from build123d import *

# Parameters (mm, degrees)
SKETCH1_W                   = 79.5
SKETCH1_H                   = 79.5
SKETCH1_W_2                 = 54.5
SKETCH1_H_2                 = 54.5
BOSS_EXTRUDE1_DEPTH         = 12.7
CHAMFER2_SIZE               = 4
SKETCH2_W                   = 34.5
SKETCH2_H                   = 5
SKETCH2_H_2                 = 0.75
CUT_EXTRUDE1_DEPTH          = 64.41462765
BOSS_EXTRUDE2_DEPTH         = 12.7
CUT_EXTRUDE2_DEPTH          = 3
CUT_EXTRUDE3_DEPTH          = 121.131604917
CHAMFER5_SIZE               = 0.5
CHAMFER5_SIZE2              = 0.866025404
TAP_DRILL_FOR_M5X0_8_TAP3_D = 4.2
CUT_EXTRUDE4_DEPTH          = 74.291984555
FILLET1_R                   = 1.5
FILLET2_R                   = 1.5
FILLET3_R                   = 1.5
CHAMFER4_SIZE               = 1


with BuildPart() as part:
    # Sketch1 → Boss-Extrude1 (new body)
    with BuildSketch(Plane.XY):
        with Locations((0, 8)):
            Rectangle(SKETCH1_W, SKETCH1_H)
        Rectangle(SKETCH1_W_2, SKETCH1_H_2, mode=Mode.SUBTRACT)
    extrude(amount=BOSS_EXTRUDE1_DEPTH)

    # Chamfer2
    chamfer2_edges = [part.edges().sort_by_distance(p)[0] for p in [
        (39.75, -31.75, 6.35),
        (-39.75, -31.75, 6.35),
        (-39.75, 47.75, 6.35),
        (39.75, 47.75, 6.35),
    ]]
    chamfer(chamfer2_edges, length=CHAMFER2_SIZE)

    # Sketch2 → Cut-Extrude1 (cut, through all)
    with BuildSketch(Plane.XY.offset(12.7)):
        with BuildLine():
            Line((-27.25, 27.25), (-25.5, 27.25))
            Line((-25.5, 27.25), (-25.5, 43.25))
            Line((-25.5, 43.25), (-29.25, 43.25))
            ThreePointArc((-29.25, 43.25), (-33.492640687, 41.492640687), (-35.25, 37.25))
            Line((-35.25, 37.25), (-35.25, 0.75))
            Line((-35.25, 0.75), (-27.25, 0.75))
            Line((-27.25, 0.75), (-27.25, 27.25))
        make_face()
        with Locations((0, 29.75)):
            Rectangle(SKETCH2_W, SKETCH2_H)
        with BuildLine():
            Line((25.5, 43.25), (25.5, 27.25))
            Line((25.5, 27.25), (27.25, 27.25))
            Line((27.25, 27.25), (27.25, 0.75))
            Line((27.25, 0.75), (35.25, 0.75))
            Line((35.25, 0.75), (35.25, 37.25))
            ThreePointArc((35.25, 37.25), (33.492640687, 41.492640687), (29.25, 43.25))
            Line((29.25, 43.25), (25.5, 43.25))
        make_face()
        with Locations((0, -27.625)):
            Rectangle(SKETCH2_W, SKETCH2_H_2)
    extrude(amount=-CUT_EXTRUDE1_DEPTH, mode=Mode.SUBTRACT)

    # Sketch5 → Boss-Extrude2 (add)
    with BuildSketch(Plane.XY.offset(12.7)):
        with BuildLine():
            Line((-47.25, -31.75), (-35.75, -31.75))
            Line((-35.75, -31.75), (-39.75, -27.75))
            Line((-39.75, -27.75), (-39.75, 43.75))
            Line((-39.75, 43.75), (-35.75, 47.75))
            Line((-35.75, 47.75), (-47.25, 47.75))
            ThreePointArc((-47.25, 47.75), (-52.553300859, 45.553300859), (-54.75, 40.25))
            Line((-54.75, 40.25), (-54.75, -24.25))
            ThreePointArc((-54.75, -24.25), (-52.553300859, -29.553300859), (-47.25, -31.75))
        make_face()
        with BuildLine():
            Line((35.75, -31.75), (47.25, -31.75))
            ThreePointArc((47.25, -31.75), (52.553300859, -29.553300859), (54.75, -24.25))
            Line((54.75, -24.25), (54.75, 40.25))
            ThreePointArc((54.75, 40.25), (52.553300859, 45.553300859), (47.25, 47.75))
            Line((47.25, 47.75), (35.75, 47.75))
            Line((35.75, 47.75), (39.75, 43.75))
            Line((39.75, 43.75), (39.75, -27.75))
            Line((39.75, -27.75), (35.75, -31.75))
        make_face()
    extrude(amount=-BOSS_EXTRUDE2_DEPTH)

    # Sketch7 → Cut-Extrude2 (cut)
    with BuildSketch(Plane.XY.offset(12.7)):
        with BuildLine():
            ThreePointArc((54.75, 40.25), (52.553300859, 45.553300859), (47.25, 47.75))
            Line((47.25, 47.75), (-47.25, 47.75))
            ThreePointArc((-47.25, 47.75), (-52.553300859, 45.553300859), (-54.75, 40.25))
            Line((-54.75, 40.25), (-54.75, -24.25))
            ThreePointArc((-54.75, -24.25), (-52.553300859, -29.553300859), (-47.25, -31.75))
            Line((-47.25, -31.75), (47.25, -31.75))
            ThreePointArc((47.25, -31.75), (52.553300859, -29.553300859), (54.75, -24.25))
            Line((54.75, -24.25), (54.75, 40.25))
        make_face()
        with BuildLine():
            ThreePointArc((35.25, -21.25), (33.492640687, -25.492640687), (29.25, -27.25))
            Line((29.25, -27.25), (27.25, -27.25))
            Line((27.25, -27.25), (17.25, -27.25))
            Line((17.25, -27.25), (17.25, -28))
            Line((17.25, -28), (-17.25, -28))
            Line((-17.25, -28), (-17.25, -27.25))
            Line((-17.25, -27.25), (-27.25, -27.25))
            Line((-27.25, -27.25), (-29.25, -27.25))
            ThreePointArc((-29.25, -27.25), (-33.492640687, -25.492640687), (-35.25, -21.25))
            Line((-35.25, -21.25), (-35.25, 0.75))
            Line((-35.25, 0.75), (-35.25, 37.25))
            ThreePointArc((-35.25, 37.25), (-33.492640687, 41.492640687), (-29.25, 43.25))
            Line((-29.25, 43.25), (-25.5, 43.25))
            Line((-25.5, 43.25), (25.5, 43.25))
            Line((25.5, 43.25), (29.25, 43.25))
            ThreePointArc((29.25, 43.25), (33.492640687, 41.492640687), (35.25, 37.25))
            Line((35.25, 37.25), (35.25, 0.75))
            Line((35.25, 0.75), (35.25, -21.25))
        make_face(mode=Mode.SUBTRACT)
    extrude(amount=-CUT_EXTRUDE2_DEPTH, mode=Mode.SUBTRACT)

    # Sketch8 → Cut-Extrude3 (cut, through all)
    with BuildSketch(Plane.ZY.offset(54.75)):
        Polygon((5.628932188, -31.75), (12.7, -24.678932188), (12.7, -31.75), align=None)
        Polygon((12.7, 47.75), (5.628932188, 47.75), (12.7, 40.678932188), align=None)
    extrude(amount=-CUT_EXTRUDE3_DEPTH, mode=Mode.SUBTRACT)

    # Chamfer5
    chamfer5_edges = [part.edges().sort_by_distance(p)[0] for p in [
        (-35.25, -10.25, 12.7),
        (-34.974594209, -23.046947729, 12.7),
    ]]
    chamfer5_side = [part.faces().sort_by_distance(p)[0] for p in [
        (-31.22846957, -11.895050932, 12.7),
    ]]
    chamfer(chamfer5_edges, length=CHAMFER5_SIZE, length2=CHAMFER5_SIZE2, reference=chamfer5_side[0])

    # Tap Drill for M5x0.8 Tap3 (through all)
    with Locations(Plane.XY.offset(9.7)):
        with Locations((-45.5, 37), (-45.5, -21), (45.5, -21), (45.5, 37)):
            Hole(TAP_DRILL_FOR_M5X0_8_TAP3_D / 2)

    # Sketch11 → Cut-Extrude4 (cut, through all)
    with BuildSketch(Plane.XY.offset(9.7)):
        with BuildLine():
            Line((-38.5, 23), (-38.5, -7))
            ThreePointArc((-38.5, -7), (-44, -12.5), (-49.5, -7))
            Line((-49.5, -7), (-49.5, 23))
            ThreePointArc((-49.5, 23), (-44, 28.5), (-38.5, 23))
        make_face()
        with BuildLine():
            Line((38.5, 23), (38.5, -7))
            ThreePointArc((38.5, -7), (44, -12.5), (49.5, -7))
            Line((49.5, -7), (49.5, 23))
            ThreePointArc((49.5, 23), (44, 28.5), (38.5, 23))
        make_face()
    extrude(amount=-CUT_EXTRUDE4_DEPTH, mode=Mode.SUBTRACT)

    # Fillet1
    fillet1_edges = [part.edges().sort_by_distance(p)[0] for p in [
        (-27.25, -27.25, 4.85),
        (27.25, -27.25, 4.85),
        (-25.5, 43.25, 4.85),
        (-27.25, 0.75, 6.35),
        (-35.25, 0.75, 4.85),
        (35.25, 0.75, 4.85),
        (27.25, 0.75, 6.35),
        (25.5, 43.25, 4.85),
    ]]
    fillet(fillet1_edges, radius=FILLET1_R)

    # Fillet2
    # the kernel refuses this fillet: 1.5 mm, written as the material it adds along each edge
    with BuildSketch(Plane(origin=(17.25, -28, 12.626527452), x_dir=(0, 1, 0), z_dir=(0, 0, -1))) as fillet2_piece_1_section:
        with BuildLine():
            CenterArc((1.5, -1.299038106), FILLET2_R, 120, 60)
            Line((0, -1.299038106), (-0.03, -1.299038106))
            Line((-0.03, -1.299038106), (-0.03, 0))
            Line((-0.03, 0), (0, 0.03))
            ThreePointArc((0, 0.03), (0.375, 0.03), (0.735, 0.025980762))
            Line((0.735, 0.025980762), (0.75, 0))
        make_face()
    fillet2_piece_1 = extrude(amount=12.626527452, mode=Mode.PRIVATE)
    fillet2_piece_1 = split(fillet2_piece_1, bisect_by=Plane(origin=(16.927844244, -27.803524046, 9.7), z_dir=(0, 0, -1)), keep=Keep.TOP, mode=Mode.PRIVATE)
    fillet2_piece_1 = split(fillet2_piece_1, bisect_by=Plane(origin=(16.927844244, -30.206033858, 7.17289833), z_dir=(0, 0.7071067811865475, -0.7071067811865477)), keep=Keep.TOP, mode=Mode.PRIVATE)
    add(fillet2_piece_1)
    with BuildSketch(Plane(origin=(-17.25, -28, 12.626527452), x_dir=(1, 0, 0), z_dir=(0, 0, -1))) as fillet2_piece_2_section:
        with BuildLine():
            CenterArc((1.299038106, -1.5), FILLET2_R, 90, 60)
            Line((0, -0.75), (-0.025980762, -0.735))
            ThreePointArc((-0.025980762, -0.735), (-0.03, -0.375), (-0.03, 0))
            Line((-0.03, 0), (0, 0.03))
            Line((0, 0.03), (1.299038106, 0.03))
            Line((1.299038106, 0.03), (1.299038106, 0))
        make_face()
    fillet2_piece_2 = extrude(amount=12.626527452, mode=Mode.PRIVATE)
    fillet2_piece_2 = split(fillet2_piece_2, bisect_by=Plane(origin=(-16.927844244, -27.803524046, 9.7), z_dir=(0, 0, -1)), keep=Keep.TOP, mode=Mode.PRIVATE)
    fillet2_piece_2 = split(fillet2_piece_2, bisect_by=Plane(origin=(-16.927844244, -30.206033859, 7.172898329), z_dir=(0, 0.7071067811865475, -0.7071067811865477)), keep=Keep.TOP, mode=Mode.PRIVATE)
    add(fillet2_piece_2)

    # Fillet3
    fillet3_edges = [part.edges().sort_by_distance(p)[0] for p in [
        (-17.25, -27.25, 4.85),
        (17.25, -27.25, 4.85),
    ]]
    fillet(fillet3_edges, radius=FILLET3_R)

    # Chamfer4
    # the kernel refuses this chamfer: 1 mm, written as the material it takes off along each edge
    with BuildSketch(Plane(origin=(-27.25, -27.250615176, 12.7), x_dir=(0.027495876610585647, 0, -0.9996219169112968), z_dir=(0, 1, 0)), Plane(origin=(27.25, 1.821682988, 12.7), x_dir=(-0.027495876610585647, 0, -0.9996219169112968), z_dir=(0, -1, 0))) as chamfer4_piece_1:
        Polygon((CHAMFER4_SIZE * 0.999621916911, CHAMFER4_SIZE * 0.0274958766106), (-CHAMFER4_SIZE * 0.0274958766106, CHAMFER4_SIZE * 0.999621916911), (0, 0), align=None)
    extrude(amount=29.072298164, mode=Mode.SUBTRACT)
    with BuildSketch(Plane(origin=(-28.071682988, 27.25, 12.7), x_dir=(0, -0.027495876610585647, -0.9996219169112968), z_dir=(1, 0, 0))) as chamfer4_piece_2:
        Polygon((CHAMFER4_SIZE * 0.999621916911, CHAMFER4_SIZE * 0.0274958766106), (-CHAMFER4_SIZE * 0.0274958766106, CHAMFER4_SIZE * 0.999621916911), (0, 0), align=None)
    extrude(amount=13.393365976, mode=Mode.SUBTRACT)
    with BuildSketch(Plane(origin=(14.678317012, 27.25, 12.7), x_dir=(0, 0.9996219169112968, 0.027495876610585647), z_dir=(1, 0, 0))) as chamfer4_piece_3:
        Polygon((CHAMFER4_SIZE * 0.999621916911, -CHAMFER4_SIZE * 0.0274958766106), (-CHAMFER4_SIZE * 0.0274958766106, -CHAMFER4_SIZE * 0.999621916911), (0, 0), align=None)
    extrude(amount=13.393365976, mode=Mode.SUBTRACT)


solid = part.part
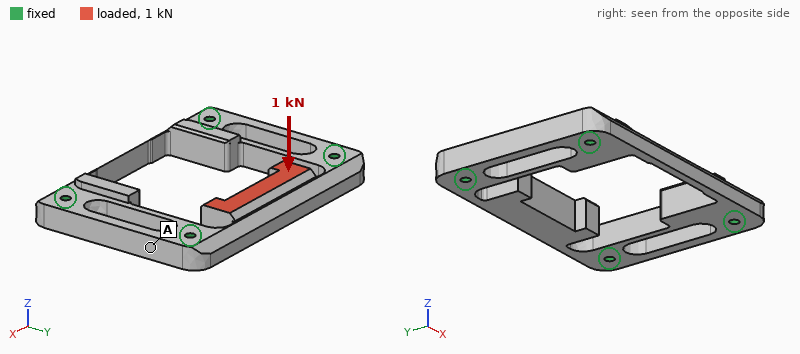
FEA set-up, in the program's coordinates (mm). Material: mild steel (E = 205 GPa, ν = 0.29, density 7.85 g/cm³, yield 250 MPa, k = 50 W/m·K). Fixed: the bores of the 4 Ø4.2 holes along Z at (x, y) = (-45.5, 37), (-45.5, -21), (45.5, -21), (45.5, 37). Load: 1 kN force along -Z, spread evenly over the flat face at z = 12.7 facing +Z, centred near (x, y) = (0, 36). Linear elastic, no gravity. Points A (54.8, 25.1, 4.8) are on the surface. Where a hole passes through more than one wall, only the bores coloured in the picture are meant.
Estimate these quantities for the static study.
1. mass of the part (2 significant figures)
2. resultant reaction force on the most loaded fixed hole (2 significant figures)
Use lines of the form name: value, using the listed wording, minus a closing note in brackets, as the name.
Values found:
mass of the part: 300 g
resultant reaction force on the most loaded fixed hole: 500 N
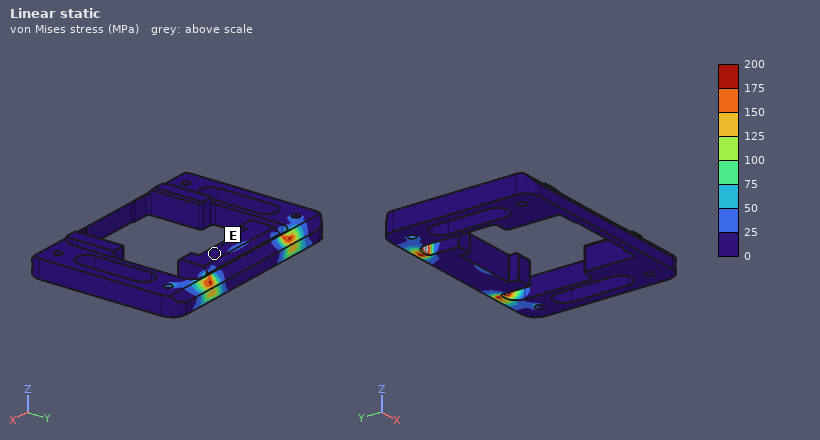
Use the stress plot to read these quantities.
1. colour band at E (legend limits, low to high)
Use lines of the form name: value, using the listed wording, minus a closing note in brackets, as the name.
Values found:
colour band at E: 0 to 25 MPa
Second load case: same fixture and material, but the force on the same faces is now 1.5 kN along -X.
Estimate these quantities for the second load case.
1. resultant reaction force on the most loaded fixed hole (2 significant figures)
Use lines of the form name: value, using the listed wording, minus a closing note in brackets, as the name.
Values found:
resultant reaction force on the most loaded fixed hole: 820 N
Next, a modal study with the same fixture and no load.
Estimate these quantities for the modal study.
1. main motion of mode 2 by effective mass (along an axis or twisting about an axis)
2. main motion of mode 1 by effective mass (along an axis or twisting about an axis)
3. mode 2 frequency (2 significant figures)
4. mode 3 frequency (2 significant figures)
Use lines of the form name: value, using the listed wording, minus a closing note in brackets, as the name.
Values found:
main motion of mode 2 by effective mass: along Y
main motion of mode 1 by effective mass: along Z
mode 2 frequency: 5000 Hz
mode 3 frequency: 6200 Hz
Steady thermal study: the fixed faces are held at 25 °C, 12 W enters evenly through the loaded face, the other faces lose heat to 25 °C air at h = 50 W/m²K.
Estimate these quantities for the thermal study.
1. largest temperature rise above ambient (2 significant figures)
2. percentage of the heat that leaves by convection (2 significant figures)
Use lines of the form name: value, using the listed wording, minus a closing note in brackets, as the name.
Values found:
largest temperature rise above ambient: 38 K
percentage of the heat that leaves by convection: 45 %
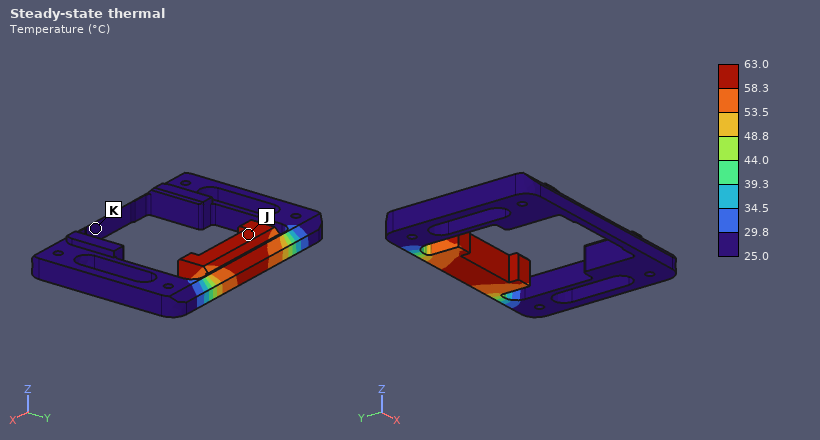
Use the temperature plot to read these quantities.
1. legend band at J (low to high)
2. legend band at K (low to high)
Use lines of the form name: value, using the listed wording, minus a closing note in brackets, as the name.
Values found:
legend band at J: 58.3 to 63.0 °C
legend band at K: 25.0 to 29.8 °C
